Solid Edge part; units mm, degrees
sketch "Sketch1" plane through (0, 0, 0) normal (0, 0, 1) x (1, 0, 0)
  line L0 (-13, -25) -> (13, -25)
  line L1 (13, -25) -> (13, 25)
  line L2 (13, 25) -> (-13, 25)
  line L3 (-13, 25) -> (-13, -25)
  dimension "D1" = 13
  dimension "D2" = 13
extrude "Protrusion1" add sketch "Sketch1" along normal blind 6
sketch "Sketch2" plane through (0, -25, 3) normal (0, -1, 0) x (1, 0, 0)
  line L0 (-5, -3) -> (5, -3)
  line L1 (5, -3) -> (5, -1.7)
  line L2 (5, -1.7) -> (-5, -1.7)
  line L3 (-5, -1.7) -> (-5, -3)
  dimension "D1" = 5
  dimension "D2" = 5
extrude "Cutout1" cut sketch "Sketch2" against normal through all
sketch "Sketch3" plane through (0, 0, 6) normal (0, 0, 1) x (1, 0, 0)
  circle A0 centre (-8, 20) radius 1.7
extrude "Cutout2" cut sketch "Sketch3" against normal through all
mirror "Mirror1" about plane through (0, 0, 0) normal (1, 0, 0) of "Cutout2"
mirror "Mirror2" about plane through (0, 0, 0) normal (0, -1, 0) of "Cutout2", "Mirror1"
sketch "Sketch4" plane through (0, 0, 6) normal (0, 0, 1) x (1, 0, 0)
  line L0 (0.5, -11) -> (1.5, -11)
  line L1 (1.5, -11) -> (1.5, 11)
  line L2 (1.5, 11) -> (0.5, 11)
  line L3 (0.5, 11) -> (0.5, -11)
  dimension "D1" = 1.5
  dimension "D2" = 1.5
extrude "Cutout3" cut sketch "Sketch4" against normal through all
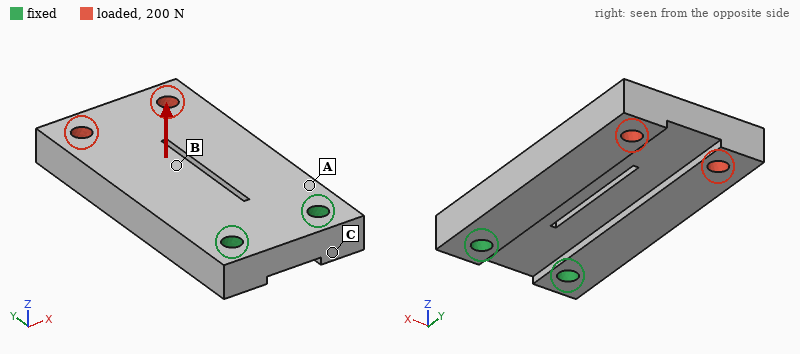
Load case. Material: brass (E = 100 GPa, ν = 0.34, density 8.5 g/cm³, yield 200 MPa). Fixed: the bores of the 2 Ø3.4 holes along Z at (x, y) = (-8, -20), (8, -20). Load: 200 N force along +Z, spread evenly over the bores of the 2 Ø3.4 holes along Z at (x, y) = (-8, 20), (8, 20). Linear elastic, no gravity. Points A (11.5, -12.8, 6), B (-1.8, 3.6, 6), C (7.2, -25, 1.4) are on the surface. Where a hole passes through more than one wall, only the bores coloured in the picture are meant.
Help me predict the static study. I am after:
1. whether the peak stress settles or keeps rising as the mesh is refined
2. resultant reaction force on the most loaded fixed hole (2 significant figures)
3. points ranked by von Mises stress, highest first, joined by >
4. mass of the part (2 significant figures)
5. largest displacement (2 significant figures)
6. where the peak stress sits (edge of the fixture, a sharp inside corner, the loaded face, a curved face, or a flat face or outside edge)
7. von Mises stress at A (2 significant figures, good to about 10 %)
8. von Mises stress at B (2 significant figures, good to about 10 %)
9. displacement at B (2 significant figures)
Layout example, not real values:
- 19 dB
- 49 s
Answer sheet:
- keeps rising
- 110 N
- A > B > C
- 58 g
- 0.13 mm
- edge of the fixture
- 48 MPa
- 24 MPa
- 0.047 mm
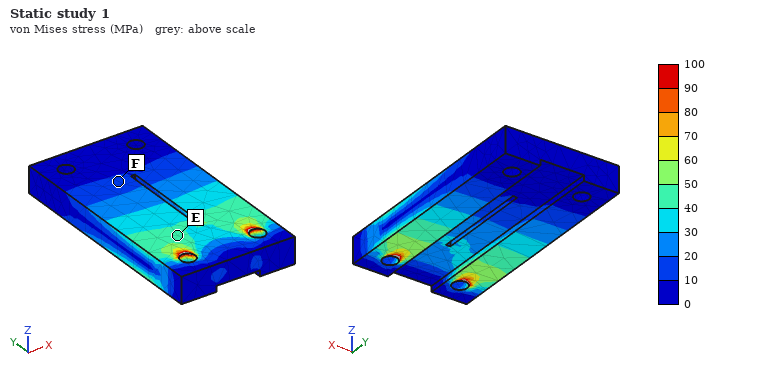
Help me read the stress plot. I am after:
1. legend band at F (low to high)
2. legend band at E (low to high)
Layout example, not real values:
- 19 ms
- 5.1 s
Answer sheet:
- 10 to 20 MPa
- 40 to 50 MPa
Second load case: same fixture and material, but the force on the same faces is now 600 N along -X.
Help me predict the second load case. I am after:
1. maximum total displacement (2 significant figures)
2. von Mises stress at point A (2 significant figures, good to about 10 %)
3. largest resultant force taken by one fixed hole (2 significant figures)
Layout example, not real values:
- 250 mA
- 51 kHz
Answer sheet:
- 34 µm
- 30 MPa
- 1.3 kN
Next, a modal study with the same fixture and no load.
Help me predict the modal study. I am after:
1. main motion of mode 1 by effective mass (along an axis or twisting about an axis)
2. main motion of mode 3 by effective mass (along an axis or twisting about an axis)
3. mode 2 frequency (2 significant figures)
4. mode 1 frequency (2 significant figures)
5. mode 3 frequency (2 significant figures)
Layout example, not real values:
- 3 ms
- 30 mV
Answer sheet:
- along Z
- along X
- 4700 Hz
- 1600 Hz
- 5200 Hz
